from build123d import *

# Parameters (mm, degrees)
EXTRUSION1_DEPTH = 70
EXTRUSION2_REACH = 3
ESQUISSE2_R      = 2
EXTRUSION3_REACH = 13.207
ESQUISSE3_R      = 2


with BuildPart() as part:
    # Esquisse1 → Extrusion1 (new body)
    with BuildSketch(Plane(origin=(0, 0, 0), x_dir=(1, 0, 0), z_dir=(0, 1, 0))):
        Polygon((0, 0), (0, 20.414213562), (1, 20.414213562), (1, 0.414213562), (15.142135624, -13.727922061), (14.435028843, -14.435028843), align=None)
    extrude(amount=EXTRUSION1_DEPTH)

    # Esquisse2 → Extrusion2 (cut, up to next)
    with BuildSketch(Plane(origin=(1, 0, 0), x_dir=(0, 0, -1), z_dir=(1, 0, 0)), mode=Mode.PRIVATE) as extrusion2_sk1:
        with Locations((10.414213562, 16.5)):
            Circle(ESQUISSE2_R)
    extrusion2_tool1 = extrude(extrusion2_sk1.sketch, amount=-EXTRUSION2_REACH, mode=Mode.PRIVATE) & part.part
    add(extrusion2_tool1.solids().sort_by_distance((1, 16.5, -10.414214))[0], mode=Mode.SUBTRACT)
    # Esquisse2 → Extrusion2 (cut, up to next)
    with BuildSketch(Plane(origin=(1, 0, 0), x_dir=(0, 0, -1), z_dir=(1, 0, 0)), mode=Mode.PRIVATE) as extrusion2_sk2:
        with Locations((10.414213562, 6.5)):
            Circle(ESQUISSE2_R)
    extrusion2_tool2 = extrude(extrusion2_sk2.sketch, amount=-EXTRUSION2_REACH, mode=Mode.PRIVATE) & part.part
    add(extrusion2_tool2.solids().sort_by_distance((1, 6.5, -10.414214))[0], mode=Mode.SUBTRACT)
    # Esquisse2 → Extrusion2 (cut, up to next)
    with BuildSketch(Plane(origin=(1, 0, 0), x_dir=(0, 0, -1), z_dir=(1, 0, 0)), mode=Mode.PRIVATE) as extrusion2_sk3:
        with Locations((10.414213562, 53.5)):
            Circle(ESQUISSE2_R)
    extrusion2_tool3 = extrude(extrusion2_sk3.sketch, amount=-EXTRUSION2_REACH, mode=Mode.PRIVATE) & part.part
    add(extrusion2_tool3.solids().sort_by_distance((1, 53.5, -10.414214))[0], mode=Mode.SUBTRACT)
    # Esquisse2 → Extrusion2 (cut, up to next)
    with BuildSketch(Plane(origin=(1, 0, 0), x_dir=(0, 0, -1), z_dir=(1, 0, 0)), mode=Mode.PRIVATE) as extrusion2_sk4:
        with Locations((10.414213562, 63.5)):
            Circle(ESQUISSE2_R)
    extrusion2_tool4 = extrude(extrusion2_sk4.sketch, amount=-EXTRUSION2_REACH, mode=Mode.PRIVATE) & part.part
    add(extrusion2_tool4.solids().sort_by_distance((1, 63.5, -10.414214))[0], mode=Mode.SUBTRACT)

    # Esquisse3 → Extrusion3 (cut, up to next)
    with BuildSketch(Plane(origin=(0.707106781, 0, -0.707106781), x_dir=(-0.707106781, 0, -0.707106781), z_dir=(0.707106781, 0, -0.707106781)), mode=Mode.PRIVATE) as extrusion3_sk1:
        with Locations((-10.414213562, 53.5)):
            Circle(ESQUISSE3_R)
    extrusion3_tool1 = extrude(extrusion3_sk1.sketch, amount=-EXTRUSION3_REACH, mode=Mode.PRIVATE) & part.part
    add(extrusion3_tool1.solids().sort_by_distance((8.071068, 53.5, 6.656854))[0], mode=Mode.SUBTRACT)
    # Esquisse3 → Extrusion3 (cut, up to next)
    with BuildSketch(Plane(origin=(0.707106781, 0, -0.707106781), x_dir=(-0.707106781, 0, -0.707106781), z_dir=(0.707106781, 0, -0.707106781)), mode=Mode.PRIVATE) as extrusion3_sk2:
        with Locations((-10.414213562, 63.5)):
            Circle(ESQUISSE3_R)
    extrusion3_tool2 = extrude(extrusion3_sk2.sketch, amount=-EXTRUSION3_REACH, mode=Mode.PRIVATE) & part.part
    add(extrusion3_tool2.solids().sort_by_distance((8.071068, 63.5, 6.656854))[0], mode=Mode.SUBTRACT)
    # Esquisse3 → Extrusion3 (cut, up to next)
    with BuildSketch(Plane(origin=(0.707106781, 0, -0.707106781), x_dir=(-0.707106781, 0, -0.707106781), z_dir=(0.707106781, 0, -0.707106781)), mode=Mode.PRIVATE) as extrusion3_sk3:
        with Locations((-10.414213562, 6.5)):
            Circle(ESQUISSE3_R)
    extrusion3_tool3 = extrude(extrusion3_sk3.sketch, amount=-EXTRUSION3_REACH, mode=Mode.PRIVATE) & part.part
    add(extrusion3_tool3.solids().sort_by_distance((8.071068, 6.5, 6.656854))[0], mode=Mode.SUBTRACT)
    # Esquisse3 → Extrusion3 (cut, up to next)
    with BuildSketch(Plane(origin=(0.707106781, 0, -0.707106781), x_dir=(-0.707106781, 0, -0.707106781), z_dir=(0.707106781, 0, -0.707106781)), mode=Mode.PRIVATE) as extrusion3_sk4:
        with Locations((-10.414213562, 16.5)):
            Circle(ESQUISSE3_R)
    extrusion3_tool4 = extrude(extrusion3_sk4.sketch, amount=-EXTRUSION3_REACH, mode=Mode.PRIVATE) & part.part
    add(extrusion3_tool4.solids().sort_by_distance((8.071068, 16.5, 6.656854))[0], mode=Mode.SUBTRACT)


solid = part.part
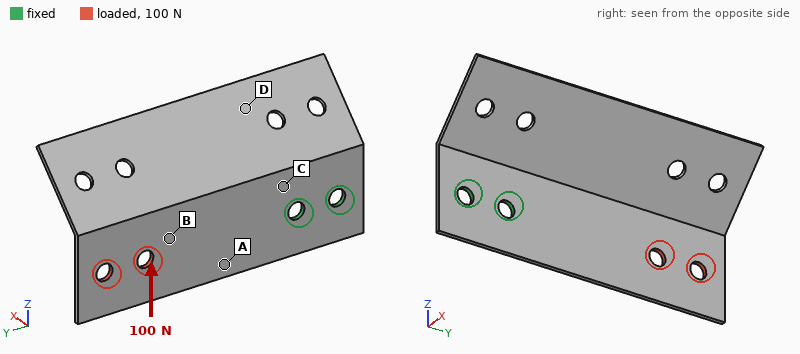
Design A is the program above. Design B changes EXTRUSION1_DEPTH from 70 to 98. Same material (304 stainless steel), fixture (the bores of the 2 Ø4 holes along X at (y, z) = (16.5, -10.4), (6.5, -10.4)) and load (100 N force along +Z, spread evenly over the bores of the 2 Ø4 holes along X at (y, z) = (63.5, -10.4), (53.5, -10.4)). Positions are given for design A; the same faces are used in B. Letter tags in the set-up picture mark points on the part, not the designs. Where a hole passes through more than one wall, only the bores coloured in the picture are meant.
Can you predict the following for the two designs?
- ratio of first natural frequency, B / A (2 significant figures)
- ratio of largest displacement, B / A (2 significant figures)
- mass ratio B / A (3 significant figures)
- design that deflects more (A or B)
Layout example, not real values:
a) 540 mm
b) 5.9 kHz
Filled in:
a) 0.58
b) 1.6
c) 1.41
d) B
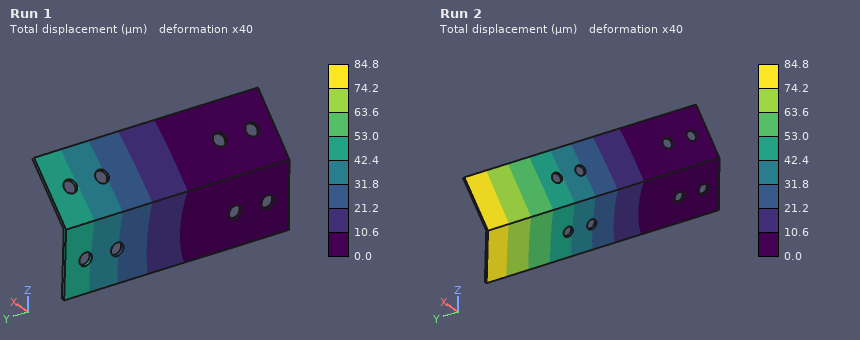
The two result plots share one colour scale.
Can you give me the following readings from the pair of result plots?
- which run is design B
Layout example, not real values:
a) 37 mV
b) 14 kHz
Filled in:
a) Run 2
